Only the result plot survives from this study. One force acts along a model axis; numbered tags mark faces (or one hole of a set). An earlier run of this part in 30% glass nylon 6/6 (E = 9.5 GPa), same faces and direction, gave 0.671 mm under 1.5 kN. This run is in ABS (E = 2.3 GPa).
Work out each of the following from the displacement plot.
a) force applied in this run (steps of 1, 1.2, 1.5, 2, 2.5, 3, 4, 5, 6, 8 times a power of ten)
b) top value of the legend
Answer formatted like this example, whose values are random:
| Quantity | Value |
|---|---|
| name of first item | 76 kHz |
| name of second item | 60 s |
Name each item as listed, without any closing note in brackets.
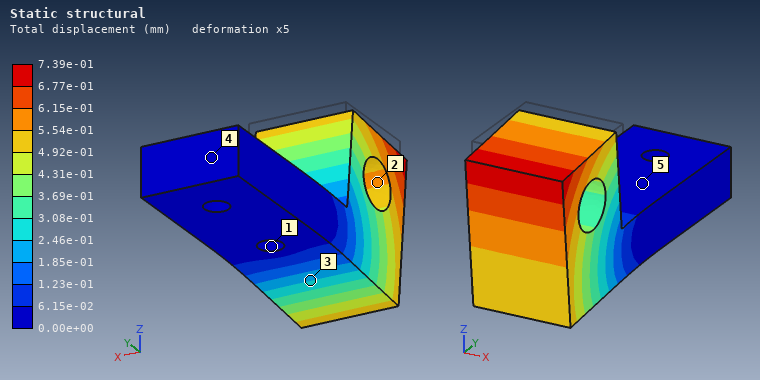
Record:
| Quantity | Value |
|---|---|
| force applied in this run | 400 N |
| top value of the legend | 7.39e-01 mm |
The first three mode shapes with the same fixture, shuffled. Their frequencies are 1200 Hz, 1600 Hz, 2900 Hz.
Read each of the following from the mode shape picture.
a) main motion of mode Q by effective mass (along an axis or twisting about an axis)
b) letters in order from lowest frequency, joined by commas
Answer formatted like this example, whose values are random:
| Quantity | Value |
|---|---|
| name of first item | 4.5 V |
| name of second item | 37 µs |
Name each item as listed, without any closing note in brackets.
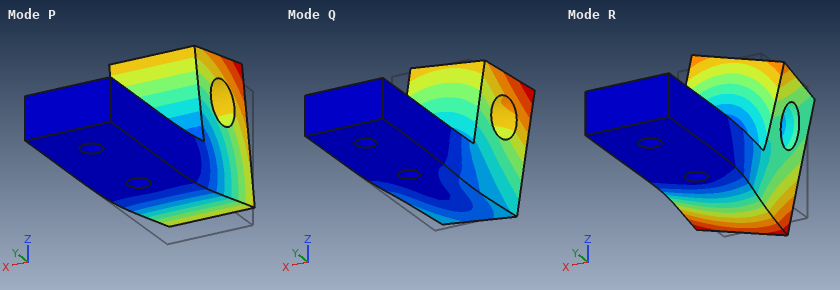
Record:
| Quantity | Value |
|---|---|
| main motion of mode Q by effective mass | along X |
| letters in order from lowest frequency, joined by commas | P, Q, R |
